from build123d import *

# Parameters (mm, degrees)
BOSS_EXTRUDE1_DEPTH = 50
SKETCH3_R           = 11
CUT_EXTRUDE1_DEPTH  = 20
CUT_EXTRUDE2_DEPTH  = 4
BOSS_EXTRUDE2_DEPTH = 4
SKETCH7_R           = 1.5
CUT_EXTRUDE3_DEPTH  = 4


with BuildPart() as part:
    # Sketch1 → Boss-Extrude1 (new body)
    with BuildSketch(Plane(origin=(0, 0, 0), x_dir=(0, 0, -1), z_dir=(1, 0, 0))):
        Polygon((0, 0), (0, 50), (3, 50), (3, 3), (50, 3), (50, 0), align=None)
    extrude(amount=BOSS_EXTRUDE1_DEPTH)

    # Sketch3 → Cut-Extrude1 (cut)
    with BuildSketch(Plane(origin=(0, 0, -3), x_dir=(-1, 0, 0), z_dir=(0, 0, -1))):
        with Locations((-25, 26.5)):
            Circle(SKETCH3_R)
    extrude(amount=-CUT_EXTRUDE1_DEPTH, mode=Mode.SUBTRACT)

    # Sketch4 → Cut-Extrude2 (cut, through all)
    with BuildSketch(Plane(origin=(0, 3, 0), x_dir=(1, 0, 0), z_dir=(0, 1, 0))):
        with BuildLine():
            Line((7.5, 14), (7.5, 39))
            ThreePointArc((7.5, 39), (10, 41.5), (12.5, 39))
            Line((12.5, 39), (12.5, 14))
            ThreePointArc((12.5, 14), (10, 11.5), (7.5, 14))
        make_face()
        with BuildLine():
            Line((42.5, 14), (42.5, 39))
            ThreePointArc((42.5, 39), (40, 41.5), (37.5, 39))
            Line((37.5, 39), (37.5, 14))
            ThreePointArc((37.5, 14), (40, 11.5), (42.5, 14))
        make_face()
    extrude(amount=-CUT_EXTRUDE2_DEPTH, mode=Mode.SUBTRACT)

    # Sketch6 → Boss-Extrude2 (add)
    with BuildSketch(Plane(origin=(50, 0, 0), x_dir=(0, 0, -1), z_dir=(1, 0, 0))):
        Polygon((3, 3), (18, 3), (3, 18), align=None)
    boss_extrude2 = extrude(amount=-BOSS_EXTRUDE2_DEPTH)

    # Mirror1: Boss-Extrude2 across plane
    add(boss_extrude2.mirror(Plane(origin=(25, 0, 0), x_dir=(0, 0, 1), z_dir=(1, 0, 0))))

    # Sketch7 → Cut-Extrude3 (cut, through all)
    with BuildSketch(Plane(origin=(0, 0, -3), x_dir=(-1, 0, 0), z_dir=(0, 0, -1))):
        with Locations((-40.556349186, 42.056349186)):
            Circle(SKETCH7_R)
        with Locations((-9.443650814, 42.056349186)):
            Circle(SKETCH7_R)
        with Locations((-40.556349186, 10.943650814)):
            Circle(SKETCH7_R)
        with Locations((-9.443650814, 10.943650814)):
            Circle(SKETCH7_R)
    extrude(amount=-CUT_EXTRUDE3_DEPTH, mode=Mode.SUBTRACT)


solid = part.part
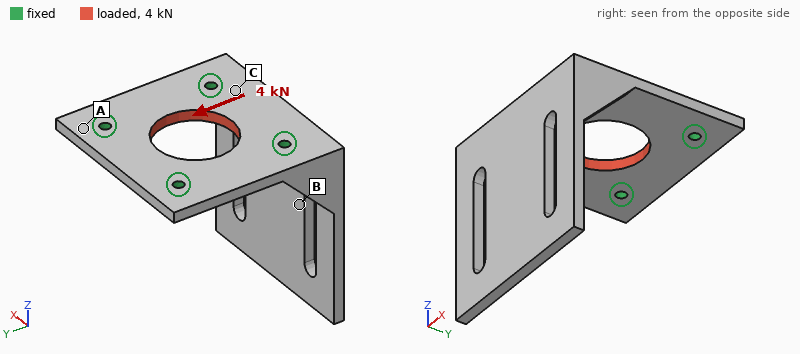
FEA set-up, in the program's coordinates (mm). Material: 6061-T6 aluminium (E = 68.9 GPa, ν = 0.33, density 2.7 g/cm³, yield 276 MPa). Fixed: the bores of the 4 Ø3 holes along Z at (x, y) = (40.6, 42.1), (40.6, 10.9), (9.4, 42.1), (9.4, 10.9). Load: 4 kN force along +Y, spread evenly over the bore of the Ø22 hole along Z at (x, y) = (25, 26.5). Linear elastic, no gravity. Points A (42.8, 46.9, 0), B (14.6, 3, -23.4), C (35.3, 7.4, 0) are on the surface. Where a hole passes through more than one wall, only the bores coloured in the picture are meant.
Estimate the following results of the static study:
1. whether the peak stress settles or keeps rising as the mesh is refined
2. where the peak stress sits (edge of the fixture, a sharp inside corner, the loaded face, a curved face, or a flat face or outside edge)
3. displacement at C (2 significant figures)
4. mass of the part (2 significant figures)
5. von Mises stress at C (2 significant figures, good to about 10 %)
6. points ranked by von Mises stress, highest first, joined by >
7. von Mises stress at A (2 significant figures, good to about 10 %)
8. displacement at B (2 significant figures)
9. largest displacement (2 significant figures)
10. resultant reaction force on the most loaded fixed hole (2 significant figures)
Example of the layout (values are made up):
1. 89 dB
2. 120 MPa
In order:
1. keeps rising
2. edge of the fixture
3. 3.4 µm
4. 36 g
5. 20 MPa
6. C > A > B
7. 10 MPa
8. 4.3 µm
9. 11 µm
10. 1.0 kN
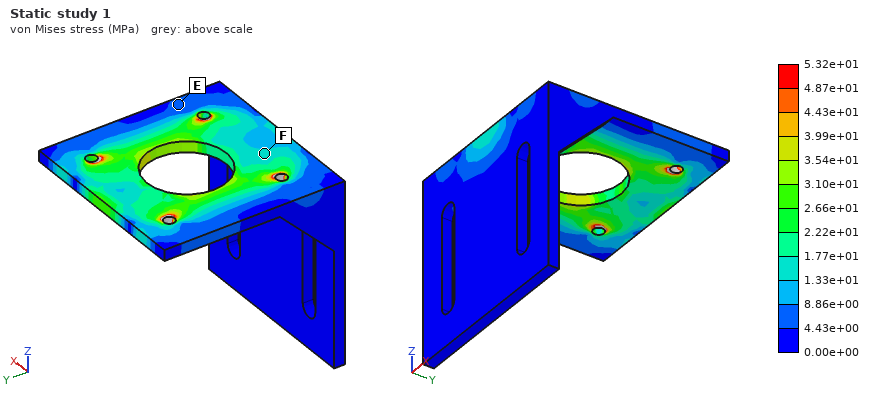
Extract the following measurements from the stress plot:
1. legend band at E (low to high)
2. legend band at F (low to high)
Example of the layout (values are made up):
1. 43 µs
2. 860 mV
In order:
1. 4.43e+00 to 8.86e+00 MPa
2. 1.33e+01 to 1.77e+01 MPa
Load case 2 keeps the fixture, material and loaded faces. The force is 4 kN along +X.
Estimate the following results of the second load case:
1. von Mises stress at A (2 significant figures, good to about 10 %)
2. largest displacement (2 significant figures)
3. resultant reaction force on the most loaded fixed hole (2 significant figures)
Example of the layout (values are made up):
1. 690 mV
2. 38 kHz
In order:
1. 8.2 MPa
2. 9.4 µm
3. 1.0 kN
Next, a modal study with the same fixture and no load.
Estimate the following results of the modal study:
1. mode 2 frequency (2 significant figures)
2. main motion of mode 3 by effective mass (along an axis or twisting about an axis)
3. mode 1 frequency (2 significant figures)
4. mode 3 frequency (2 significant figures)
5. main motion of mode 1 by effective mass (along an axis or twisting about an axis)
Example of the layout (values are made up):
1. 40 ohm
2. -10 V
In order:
1. 2600 Hz
2. along X
3. 1100 Hz
4. 4000 Hz
5. along Y
